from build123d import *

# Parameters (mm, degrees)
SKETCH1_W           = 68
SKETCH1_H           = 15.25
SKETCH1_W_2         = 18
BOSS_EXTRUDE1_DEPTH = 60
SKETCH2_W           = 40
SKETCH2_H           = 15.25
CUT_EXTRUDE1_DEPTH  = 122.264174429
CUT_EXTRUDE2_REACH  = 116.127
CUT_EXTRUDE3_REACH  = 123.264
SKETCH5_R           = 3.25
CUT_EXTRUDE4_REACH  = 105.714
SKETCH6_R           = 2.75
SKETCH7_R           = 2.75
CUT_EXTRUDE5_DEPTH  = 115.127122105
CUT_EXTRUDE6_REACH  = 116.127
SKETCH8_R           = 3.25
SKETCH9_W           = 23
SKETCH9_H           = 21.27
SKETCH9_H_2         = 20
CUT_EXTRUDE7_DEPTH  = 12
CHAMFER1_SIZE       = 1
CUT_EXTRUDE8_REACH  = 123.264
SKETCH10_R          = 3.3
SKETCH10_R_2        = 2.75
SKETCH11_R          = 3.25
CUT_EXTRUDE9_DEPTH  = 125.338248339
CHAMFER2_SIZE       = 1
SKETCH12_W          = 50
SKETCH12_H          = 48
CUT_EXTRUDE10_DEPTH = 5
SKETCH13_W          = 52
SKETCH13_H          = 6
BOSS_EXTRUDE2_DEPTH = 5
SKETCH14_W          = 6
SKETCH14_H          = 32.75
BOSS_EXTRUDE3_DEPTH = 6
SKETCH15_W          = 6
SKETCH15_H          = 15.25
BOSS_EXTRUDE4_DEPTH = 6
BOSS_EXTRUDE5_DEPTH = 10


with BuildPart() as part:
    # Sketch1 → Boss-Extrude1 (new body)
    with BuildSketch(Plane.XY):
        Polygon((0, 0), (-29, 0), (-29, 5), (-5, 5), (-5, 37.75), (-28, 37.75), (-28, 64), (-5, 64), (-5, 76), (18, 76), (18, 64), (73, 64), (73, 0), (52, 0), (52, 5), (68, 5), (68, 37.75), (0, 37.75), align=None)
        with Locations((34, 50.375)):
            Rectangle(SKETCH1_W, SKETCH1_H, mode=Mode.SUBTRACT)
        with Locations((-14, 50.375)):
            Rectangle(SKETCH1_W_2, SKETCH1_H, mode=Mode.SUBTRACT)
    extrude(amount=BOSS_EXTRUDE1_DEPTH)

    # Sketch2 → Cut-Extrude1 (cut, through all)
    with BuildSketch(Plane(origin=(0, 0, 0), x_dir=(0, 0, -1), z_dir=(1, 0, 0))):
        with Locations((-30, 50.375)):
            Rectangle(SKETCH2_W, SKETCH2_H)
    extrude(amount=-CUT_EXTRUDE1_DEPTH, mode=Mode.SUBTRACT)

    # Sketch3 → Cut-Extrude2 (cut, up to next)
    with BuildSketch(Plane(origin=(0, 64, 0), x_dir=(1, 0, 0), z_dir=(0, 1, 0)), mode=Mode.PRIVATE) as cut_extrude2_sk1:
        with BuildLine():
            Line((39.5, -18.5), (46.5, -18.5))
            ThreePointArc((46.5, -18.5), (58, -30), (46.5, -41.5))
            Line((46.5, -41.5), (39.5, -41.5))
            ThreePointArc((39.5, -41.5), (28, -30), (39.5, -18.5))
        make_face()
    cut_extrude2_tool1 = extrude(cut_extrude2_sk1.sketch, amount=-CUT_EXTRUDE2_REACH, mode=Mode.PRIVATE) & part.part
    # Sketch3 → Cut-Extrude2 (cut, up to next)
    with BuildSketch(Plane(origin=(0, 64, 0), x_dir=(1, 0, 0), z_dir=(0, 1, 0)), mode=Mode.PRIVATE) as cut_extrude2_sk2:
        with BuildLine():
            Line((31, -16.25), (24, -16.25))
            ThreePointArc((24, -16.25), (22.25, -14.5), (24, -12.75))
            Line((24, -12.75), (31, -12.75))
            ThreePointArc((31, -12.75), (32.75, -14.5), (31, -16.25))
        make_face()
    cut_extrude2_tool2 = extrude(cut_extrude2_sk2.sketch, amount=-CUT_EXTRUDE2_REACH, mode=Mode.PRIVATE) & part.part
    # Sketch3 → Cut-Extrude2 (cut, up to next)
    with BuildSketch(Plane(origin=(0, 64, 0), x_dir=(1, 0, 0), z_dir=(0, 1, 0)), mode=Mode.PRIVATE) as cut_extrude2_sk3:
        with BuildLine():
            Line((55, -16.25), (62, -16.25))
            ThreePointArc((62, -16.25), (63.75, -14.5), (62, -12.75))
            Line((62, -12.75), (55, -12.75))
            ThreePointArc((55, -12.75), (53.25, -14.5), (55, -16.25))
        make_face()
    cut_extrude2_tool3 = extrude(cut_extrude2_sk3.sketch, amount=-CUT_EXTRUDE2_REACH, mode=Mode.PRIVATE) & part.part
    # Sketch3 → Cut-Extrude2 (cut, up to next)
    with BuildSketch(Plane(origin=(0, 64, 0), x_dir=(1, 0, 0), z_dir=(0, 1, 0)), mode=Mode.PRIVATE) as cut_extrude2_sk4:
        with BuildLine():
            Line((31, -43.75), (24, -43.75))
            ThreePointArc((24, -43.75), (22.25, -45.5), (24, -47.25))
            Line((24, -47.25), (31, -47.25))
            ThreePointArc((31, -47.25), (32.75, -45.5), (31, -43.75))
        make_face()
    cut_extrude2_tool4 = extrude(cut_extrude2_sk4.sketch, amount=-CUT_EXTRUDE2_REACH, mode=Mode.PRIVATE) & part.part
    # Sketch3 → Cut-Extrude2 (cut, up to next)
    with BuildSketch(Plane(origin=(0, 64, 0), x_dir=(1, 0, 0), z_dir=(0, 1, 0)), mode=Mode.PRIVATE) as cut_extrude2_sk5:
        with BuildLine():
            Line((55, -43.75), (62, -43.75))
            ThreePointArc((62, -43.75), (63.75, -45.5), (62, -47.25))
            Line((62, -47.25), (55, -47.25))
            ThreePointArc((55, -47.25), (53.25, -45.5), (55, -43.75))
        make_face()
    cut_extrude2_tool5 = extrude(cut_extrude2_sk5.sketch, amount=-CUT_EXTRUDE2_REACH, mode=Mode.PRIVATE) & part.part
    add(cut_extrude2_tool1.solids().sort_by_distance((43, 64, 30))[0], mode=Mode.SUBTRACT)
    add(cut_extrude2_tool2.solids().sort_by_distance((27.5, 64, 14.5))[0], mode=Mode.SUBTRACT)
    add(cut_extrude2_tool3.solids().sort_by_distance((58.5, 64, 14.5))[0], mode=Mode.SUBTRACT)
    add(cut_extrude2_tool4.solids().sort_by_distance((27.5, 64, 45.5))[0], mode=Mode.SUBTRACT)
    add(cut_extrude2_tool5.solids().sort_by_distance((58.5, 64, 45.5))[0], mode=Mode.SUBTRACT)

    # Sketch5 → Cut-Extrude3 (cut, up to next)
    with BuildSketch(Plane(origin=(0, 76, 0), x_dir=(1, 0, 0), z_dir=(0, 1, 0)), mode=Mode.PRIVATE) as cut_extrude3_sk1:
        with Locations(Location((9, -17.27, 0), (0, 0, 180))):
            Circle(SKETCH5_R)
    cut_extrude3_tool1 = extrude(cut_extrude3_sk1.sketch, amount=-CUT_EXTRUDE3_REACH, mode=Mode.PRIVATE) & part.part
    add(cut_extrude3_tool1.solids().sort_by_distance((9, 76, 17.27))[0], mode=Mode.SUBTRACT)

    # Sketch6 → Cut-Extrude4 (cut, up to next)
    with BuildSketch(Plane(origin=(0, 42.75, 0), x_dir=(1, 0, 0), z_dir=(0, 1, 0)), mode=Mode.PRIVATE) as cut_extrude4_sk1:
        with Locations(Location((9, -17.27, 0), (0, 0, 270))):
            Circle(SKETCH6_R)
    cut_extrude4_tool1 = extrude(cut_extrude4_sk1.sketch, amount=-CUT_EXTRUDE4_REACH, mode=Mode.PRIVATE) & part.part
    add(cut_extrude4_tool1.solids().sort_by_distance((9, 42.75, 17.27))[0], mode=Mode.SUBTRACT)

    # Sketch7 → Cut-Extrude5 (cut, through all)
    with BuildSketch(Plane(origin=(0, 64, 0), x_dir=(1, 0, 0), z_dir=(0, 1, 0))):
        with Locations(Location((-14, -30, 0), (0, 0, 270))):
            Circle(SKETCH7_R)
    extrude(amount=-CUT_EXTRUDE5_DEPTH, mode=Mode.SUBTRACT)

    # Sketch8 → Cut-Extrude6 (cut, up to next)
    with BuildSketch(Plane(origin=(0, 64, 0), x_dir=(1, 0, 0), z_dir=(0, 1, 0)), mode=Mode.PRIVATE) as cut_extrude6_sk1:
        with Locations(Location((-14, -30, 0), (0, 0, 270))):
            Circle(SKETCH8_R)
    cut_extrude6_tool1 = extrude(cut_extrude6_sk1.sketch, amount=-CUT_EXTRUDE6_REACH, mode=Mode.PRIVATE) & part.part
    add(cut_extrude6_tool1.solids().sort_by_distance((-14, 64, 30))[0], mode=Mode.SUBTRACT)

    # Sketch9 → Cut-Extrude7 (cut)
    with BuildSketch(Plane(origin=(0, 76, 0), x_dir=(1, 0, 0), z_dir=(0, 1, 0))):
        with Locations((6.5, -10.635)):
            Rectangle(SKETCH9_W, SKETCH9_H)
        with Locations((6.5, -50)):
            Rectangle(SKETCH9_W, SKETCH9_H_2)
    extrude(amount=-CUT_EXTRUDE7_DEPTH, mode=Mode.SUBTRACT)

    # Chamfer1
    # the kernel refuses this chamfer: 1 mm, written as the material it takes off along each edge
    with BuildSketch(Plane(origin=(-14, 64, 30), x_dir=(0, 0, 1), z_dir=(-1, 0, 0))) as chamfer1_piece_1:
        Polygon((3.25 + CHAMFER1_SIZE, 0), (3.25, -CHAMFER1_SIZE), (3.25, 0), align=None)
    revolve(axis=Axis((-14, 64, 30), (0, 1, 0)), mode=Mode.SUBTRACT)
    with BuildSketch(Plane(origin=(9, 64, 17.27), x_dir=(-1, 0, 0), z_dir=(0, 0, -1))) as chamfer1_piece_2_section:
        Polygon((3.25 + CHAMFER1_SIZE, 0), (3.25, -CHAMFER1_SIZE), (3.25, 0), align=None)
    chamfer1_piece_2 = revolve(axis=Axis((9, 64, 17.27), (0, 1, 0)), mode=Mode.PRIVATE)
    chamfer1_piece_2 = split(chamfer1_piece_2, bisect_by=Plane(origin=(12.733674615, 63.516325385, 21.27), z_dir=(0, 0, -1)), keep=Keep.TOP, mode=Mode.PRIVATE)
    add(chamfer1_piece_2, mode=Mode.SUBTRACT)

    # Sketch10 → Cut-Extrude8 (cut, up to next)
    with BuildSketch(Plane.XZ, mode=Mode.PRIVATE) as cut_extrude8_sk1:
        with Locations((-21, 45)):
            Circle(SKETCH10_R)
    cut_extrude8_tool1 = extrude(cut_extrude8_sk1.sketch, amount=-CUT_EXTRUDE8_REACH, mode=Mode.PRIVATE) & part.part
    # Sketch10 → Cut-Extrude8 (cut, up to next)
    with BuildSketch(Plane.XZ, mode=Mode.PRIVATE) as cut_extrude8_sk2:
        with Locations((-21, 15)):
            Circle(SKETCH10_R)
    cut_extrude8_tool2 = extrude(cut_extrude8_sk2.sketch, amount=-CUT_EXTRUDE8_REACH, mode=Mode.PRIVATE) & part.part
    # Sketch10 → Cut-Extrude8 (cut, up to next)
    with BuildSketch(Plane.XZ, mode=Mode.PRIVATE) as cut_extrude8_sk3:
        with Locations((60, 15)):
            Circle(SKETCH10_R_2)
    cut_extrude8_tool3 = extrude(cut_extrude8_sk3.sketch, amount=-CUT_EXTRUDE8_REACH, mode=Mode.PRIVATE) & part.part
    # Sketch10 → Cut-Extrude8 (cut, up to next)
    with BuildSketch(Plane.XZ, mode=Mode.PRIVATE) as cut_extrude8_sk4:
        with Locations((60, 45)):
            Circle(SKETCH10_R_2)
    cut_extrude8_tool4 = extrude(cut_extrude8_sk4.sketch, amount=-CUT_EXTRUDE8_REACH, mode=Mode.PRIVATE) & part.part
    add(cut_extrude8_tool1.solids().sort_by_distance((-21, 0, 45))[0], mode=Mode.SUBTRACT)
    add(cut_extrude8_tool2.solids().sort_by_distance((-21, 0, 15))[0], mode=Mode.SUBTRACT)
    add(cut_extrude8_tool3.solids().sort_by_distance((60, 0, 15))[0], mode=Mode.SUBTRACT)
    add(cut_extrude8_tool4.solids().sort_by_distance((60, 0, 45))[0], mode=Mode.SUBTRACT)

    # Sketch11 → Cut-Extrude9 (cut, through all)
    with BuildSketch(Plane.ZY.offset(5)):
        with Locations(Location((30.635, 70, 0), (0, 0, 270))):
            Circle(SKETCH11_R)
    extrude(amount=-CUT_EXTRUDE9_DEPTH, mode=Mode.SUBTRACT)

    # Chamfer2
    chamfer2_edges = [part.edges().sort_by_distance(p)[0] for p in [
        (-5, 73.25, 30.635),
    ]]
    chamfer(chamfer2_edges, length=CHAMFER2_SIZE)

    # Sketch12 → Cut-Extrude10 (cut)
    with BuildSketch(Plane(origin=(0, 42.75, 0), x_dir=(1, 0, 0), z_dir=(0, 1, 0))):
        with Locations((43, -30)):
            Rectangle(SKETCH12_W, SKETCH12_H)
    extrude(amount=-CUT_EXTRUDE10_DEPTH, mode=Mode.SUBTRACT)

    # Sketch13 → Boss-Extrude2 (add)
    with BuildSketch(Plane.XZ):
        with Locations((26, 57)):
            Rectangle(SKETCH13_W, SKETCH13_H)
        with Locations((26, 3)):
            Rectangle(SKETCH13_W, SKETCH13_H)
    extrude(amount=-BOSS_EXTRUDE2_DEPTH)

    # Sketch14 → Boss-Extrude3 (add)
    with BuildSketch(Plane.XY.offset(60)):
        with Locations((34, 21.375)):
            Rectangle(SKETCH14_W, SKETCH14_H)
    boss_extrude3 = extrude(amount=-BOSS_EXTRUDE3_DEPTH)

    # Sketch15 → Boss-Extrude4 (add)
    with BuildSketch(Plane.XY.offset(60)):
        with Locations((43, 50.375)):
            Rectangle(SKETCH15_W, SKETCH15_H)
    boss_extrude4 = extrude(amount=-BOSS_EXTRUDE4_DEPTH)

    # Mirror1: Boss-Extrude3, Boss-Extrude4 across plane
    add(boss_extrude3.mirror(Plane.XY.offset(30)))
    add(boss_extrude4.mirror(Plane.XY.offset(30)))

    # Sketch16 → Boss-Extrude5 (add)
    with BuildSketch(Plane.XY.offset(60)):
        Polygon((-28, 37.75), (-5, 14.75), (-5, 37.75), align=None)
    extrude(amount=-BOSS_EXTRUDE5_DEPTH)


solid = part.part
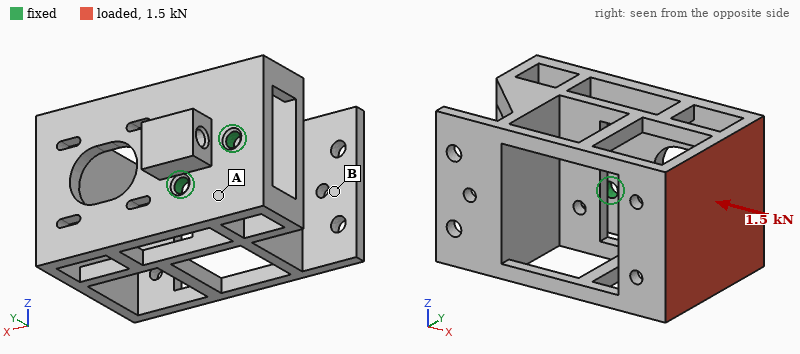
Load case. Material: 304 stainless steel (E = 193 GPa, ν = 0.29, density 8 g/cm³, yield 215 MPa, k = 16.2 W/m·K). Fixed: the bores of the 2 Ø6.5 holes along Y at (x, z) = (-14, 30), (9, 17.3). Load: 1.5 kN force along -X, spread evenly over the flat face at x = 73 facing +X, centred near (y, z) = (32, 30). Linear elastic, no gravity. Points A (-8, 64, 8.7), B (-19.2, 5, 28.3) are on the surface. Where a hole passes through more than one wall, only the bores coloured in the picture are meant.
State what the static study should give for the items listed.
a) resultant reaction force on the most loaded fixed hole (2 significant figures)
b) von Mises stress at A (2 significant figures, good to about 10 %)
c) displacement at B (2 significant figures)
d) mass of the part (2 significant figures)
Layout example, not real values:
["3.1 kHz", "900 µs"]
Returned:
["1.3 kN", "15 MPa", "0.083 mm", "840 g"]
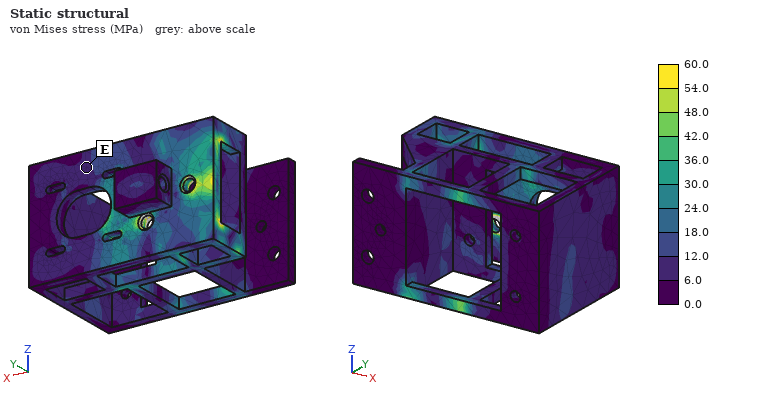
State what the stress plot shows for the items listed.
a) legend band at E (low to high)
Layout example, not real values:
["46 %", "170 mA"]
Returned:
["6.0 to 12.0 MPa"]
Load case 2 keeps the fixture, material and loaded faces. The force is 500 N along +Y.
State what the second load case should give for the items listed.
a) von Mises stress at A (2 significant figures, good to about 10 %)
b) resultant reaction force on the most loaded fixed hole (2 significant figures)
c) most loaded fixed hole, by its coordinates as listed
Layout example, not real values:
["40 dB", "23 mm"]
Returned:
["12 MPa", "1.1 kN", "(9, 17.3)"]
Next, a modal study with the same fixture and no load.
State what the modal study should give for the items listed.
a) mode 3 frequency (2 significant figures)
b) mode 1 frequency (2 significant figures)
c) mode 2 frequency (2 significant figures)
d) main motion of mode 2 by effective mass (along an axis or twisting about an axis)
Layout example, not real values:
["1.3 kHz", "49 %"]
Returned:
["1600 Hz", "620 Hz", "890 Hz", "along Z"]
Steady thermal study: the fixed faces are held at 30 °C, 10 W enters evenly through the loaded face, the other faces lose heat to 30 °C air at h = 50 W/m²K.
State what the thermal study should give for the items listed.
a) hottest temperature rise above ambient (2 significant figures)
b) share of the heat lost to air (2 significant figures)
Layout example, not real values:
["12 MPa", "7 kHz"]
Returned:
["23 K", "97 %"]
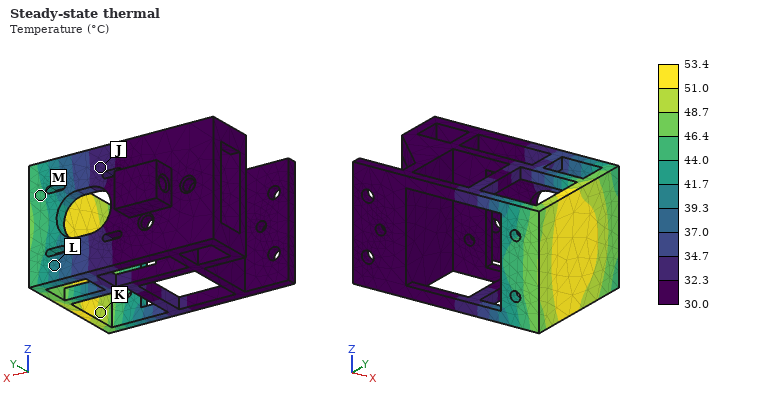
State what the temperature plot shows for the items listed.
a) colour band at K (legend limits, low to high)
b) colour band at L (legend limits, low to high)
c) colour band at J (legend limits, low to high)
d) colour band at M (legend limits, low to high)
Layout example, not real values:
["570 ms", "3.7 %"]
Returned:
["48.7 to 51.0 °C", "39.3 to 41.7 °C", "32.3 to 34.7 °C", "44.0 to 46.4 °C"]
